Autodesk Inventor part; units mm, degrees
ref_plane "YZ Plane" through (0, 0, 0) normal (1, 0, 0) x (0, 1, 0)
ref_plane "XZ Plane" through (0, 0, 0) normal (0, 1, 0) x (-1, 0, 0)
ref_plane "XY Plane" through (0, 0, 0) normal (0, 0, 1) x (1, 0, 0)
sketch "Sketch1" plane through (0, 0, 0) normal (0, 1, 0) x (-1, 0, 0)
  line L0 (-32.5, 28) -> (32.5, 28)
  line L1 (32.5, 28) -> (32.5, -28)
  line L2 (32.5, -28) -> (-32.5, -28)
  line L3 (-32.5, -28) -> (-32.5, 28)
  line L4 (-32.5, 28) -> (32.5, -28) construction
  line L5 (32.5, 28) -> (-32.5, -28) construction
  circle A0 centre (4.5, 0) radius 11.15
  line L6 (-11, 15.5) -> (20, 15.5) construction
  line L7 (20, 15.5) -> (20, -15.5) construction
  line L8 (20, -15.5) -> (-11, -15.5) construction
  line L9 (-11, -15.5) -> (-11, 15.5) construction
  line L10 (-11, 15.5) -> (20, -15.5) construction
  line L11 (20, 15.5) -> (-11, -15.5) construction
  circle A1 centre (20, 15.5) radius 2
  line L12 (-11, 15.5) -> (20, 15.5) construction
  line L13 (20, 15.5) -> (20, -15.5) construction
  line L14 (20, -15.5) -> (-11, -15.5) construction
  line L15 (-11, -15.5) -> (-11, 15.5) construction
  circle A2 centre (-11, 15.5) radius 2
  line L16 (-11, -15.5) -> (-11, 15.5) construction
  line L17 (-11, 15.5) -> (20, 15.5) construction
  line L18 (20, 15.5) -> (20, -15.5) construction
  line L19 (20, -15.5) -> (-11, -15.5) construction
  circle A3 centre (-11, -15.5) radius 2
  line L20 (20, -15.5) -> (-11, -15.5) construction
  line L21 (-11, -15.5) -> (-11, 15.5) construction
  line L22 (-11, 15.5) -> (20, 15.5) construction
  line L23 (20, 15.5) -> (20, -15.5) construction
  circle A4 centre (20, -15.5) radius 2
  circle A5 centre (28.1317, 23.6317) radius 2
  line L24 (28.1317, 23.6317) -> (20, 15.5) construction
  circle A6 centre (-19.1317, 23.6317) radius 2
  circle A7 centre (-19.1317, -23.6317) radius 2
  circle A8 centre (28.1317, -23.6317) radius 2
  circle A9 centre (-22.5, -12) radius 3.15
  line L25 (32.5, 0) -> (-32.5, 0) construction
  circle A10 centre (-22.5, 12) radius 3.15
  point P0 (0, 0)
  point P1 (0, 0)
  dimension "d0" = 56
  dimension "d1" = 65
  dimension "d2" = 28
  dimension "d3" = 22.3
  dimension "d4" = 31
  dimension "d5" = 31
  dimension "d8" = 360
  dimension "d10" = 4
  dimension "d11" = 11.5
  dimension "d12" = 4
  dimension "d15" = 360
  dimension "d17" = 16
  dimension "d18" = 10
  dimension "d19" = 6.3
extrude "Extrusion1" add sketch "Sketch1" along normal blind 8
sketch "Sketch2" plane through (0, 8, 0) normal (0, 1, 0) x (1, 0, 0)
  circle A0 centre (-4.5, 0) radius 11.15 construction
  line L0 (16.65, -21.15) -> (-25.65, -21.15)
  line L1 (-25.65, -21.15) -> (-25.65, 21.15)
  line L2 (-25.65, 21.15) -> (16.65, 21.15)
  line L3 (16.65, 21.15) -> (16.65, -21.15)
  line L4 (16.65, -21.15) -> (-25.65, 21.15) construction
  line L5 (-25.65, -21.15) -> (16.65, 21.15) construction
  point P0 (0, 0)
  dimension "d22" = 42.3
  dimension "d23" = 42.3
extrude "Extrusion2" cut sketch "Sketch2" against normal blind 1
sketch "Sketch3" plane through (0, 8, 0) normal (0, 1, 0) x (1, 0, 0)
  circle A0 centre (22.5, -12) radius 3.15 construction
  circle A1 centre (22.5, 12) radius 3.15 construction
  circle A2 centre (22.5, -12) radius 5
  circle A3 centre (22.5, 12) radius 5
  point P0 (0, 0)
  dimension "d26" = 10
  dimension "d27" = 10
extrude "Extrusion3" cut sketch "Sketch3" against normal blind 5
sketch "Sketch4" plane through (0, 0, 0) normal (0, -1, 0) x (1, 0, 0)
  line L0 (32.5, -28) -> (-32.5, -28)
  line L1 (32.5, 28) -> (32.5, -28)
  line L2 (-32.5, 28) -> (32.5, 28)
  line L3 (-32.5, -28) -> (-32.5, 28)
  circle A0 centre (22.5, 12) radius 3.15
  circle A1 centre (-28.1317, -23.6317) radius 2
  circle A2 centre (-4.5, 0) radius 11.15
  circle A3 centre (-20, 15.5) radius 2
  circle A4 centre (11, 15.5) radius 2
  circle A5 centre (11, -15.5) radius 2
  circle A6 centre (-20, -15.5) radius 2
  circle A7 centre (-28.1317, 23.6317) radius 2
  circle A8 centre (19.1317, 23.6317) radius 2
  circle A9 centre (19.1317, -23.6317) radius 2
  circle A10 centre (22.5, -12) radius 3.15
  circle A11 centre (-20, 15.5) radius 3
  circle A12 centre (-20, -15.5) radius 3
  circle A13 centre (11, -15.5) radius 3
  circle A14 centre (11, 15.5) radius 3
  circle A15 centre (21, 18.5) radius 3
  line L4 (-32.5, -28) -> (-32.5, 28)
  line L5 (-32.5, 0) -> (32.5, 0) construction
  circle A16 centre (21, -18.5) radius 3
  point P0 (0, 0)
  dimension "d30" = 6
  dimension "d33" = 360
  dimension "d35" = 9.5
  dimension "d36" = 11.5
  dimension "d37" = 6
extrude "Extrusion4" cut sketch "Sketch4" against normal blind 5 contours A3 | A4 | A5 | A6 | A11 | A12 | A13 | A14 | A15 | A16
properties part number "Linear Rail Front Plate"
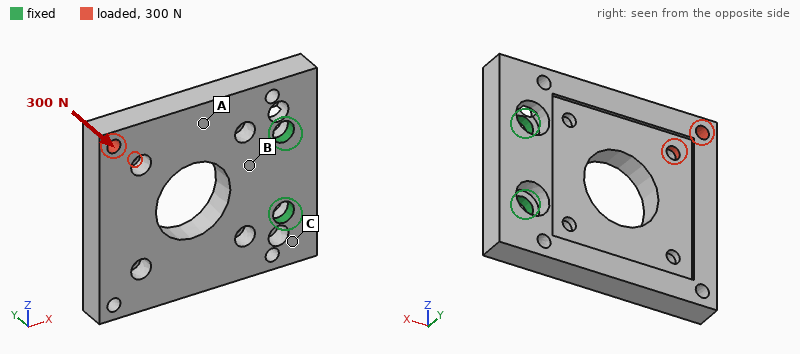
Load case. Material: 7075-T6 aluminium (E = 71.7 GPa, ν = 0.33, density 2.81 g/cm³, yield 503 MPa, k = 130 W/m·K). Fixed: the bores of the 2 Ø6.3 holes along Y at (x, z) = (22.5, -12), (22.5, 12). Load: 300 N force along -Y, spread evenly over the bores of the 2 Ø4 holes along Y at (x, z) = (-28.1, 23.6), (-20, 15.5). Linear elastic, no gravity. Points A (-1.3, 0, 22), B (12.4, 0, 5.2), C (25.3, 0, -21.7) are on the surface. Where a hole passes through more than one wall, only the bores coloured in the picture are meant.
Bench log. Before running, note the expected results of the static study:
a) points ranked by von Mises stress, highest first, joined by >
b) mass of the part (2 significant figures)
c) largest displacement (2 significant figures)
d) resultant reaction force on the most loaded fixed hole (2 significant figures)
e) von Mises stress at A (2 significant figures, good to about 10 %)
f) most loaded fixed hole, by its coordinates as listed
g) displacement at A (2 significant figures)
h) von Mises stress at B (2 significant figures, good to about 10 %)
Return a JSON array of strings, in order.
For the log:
["B > A > C", "63 g", "0.32 mm", "410 N", "25 MPa", "(22.5, 12)", "0.10 mm", "40 MPa"]
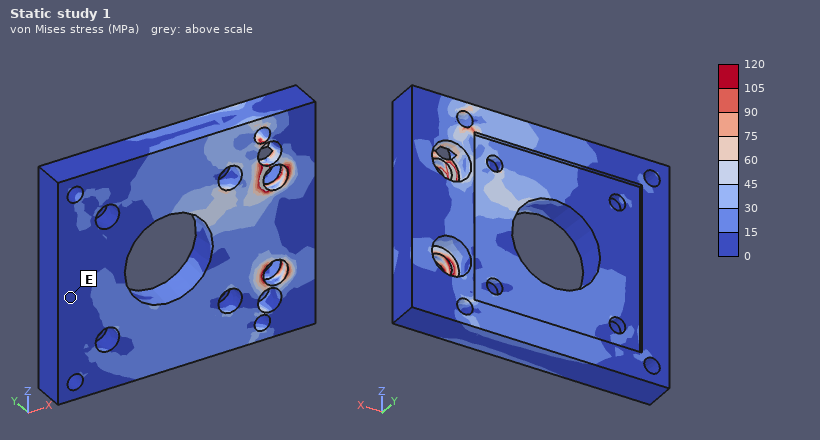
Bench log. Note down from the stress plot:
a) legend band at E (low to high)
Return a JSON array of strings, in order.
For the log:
["0 to 15 MPa"]
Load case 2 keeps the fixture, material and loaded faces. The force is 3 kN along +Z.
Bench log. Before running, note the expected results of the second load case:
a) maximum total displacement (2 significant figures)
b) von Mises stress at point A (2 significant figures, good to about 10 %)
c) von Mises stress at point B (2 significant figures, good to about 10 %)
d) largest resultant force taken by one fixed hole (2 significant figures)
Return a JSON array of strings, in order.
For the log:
["0.15 mm", "32 MPa", "65 MPa", "5.6 kN"]
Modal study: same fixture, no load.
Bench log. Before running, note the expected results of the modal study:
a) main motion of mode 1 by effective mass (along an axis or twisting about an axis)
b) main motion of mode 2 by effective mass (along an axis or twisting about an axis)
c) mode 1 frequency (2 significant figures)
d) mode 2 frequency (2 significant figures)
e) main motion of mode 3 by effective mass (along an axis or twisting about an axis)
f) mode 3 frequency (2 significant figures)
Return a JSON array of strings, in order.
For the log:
["along Y", "twisting about X", "1300 Hz", "3200 Hz", "along Z", "5000 Hz"]
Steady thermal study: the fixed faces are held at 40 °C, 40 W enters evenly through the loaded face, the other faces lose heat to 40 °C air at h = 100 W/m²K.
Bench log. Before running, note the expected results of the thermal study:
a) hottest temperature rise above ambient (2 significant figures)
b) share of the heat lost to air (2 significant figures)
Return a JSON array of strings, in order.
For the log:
["70 K", "46 %"]
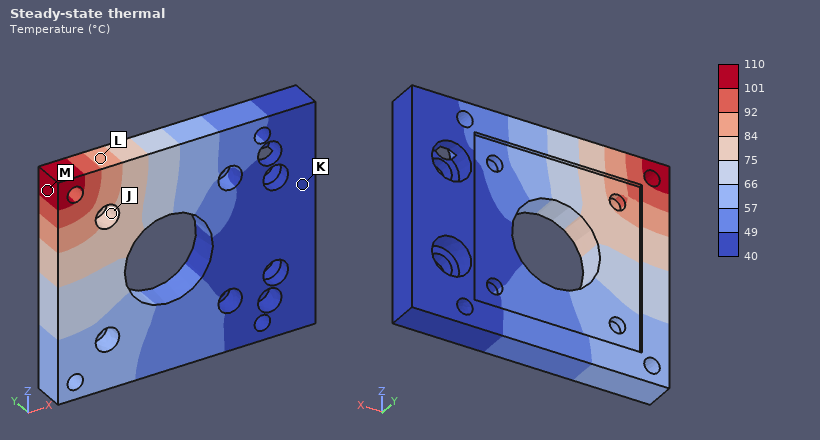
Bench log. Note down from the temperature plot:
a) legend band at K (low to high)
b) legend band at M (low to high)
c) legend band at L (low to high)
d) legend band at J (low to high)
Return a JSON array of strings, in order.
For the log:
["40 to 49 °C", "101 to 110 °C", "84 to 92 °C", "75 to 84 °C"]
